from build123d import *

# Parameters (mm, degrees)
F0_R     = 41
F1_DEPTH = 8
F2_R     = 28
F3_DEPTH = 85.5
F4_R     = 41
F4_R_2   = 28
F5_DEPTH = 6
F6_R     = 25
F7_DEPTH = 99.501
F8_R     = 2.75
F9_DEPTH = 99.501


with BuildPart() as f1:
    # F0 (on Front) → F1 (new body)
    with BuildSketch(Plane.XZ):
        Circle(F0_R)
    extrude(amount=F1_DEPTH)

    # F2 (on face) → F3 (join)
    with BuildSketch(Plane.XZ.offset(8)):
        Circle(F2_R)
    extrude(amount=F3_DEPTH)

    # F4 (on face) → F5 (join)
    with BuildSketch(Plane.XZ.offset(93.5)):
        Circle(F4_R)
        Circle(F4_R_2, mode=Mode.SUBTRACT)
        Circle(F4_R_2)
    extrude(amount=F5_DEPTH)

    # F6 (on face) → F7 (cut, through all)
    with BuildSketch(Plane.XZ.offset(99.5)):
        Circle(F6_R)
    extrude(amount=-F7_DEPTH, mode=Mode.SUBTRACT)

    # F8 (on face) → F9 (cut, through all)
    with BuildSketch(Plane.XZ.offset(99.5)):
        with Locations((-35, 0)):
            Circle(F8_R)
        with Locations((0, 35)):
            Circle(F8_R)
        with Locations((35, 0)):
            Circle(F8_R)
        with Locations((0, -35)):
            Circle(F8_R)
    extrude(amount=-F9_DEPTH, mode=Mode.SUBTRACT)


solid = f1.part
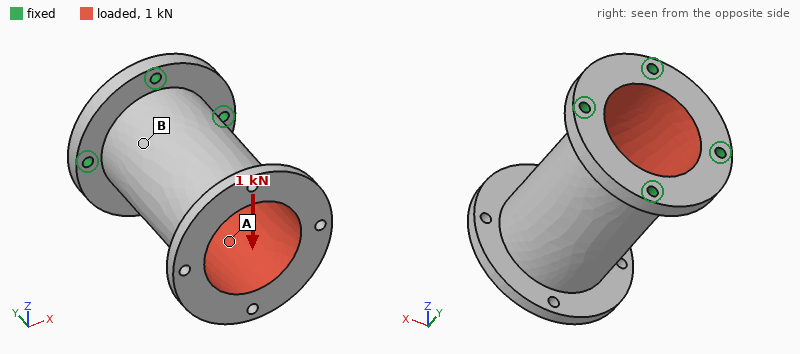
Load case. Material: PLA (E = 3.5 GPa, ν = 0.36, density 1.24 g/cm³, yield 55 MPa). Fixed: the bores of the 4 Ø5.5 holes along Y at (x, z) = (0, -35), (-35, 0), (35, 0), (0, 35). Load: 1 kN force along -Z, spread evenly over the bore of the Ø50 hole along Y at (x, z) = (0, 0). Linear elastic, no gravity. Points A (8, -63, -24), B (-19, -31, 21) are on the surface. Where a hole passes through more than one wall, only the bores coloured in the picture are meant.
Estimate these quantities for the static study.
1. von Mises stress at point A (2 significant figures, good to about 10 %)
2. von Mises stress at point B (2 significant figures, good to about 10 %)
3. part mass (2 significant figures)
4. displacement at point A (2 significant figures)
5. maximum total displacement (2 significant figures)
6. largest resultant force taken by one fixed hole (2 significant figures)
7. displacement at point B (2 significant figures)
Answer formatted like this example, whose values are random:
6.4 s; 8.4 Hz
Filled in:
1.8 MPa; 4.4 MPa; 110 g; 0.35 mm; 0.55 mm; 750 N; 0.18 mm
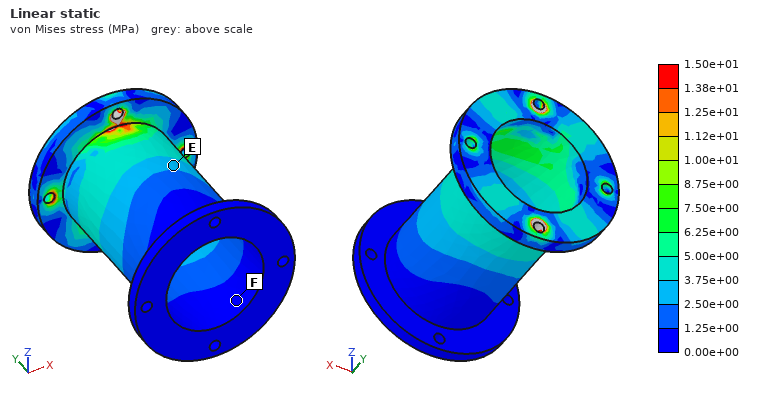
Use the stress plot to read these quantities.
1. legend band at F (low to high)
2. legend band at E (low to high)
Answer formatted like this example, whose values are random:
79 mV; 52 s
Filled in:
0.00e+00 to 1.25e+00 MPa; 2.50e+00 to 3.75e+00 MPa
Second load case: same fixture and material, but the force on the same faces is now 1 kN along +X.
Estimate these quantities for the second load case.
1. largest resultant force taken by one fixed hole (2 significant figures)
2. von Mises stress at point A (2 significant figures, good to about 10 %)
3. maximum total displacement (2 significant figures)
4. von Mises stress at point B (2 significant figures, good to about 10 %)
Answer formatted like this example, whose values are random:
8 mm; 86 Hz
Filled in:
750 N; 2.4 MPa; 0.55 mm; 4.4 MPa
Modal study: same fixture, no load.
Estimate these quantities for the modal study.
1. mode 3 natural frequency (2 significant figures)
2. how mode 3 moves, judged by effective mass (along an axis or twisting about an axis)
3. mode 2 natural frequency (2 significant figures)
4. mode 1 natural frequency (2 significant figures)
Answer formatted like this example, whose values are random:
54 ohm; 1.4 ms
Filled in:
1700 Hz; twisting about Y; 730 Hz; 730 Hz
